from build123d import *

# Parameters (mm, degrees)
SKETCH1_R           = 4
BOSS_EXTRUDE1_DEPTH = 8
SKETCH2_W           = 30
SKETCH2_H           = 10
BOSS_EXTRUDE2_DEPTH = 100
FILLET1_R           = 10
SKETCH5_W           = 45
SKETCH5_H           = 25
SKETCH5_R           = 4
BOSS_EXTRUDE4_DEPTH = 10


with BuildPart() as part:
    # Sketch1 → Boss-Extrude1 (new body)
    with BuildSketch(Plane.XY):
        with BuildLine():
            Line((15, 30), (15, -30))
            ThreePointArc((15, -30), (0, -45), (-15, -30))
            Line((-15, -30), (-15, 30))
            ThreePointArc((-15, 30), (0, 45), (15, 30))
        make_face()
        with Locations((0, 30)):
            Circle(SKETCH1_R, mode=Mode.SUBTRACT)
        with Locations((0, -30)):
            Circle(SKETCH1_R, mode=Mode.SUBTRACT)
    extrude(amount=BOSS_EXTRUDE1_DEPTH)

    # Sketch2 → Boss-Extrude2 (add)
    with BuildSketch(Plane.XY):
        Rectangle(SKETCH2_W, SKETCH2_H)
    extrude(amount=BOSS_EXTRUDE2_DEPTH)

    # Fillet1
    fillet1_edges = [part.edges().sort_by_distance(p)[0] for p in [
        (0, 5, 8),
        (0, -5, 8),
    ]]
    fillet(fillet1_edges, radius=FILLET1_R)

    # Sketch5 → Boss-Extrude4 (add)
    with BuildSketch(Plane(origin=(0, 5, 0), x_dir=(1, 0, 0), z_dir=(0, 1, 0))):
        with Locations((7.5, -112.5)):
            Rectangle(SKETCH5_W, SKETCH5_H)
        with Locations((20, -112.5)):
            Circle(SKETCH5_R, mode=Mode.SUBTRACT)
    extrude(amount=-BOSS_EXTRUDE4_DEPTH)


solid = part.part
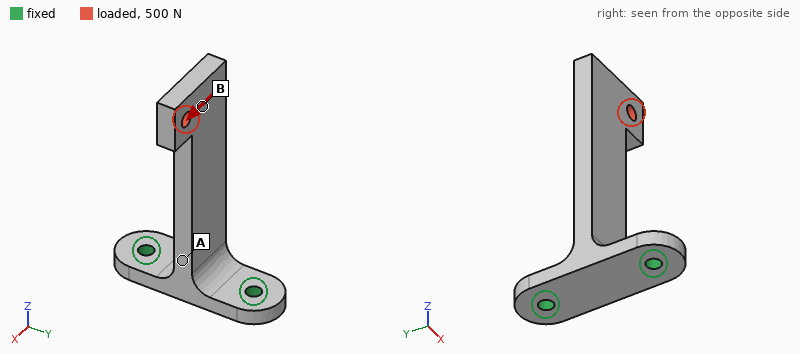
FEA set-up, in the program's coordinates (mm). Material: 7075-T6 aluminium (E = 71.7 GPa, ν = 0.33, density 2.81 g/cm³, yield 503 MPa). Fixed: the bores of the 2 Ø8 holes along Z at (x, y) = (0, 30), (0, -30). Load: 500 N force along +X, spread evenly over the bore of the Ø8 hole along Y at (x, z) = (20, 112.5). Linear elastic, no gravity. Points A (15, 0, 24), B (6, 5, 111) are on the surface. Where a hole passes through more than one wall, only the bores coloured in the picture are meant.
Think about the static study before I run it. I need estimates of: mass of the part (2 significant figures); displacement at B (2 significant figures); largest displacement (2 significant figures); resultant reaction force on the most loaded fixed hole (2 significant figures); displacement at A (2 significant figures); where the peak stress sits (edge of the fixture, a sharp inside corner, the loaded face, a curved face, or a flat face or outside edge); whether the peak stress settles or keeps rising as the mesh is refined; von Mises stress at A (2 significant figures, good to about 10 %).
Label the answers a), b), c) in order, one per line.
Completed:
a) 170 g
b) 0.52 mm
c) 0.61 mm
d) 250 N
e) 0.10 mm
f) edge of the fixture
g) keeps rising
h) 30 MPa
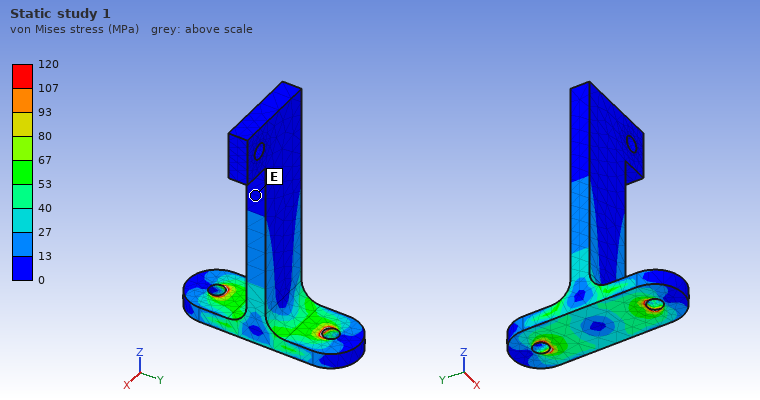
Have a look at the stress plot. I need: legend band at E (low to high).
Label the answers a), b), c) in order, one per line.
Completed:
a) 0 to 13 MPa
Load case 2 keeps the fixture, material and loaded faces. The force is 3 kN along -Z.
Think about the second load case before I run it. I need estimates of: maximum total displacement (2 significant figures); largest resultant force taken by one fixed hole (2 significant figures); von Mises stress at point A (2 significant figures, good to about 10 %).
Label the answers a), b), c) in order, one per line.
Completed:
a) 0.79 mm
b) 1.6 kN
c) 50 MPa
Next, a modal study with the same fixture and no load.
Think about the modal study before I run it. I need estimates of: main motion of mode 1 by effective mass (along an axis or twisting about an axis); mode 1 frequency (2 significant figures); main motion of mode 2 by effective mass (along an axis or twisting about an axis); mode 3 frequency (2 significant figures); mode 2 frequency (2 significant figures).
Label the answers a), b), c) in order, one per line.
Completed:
a) along Y
b) 530 Hz
c) along X
d) 2700 Hz
e) 690 Hz
